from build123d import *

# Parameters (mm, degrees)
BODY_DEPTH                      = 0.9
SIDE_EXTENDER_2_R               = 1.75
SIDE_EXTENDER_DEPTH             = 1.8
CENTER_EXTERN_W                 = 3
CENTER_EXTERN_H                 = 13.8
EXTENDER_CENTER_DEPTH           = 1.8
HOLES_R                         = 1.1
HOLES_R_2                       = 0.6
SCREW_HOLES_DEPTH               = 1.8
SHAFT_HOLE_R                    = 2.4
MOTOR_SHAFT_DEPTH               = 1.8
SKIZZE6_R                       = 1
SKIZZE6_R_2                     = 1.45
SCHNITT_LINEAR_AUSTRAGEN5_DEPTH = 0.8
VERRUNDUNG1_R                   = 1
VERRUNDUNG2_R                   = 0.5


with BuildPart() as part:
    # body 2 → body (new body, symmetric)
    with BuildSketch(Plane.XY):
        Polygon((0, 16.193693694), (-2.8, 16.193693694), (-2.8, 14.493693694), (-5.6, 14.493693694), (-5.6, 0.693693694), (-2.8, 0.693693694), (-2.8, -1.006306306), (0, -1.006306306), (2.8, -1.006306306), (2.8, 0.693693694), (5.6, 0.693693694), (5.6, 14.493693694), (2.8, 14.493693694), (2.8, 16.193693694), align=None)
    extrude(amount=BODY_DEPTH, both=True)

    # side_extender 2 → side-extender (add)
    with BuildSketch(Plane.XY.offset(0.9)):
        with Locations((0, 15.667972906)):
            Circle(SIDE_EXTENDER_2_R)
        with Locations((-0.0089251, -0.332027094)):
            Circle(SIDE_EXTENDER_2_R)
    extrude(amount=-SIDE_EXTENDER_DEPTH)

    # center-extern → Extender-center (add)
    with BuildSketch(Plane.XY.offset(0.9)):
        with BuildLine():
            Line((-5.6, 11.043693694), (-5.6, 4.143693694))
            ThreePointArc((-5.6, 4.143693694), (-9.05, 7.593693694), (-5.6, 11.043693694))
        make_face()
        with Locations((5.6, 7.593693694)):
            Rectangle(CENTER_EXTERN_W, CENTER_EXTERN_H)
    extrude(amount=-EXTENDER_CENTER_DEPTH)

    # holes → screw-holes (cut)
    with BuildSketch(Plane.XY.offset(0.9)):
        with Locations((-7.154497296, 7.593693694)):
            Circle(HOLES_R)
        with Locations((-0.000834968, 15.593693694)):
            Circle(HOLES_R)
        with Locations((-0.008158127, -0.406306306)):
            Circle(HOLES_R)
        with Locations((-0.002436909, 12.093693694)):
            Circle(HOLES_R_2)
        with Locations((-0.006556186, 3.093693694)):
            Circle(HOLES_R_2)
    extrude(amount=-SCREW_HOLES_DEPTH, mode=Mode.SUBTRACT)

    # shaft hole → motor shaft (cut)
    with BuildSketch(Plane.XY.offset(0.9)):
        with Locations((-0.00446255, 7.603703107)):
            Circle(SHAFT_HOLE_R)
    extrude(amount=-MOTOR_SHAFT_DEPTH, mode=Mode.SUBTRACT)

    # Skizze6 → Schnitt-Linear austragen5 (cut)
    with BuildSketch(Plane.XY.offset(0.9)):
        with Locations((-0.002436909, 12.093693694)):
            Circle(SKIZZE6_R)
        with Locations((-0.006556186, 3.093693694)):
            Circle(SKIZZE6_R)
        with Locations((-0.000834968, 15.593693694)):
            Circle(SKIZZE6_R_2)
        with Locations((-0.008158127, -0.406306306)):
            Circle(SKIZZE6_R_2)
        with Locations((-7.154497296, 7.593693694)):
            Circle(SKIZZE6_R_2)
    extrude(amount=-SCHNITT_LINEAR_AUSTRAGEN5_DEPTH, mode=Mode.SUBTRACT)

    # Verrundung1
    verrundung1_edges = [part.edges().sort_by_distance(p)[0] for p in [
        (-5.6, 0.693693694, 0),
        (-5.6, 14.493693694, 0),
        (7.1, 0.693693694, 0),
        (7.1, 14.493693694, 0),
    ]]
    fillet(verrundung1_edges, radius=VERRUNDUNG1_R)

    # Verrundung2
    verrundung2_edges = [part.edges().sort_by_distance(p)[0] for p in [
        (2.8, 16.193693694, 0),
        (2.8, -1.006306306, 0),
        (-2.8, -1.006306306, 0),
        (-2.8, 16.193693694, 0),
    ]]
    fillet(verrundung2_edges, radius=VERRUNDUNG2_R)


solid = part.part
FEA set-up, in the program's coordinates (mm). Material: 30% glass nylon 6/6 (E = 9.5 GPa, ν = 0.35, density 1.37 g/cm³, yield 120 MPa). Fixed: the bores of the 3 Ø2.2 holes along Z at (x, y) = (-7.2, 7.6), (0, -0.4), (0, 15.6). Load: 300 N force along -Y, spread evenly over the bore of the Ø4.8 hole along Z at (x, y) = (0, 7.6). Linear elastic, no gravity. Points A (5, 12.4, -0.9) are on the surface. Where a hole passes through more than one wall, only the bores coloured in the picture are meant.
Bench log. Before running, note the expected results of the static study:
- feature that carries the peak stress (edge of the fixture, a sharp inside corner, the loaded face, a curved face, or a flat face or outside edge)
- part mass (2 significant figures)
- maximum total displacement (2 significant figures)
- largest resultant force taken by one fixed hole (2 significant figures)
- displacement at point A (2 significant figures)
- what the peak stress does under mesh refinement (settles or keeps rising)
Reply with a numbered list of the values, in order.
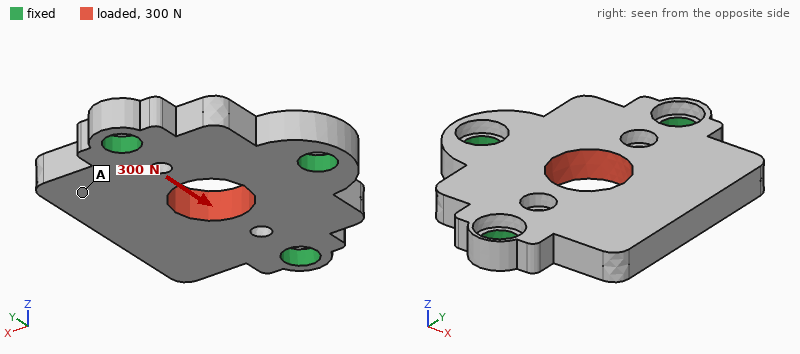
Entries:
1. edge of the fixture
2. 0.44 g
3. 14 µm
4. 130 N
5. 10 µm
6. keeps rising
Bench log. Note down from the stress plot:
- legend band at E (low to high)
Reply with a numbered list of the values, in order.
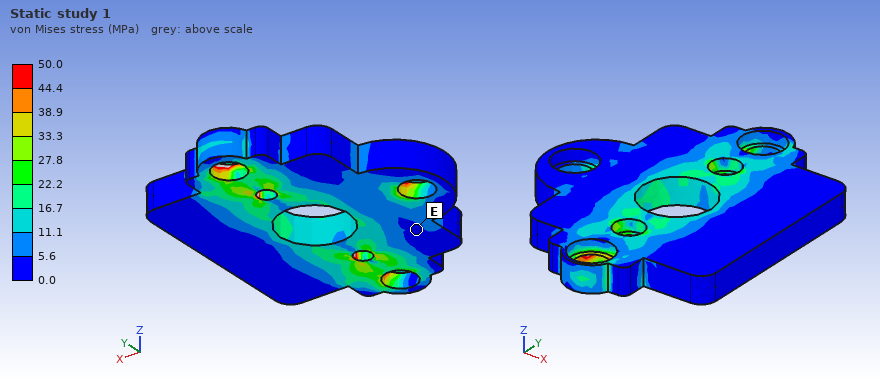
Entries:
1. 0.0 to 5.6 MPa
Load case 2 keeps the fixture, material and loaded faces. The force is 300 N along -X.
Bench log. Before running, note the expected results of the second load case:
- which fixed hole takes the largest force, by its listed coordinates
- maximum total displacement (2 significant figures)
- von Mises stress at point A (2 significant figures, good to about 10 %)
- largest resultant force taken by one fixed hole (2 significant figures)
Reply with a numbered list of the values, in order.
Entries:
1. (-7.2, 7.6)
2. 28 µm
3. 8.7 MPa
4. 150 N
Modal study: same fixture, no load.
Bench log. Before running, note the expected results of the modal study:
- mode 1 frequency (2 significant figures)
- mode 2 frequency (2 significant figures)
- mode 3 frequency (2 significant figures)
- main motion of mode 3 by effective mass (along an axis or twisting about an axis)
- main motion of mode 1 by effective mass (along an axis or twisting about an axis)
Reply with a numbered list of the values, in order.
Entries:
1. 8500 Hz
2. 20 kHz
3. 28 kHz
4. along Z
5. along Z
